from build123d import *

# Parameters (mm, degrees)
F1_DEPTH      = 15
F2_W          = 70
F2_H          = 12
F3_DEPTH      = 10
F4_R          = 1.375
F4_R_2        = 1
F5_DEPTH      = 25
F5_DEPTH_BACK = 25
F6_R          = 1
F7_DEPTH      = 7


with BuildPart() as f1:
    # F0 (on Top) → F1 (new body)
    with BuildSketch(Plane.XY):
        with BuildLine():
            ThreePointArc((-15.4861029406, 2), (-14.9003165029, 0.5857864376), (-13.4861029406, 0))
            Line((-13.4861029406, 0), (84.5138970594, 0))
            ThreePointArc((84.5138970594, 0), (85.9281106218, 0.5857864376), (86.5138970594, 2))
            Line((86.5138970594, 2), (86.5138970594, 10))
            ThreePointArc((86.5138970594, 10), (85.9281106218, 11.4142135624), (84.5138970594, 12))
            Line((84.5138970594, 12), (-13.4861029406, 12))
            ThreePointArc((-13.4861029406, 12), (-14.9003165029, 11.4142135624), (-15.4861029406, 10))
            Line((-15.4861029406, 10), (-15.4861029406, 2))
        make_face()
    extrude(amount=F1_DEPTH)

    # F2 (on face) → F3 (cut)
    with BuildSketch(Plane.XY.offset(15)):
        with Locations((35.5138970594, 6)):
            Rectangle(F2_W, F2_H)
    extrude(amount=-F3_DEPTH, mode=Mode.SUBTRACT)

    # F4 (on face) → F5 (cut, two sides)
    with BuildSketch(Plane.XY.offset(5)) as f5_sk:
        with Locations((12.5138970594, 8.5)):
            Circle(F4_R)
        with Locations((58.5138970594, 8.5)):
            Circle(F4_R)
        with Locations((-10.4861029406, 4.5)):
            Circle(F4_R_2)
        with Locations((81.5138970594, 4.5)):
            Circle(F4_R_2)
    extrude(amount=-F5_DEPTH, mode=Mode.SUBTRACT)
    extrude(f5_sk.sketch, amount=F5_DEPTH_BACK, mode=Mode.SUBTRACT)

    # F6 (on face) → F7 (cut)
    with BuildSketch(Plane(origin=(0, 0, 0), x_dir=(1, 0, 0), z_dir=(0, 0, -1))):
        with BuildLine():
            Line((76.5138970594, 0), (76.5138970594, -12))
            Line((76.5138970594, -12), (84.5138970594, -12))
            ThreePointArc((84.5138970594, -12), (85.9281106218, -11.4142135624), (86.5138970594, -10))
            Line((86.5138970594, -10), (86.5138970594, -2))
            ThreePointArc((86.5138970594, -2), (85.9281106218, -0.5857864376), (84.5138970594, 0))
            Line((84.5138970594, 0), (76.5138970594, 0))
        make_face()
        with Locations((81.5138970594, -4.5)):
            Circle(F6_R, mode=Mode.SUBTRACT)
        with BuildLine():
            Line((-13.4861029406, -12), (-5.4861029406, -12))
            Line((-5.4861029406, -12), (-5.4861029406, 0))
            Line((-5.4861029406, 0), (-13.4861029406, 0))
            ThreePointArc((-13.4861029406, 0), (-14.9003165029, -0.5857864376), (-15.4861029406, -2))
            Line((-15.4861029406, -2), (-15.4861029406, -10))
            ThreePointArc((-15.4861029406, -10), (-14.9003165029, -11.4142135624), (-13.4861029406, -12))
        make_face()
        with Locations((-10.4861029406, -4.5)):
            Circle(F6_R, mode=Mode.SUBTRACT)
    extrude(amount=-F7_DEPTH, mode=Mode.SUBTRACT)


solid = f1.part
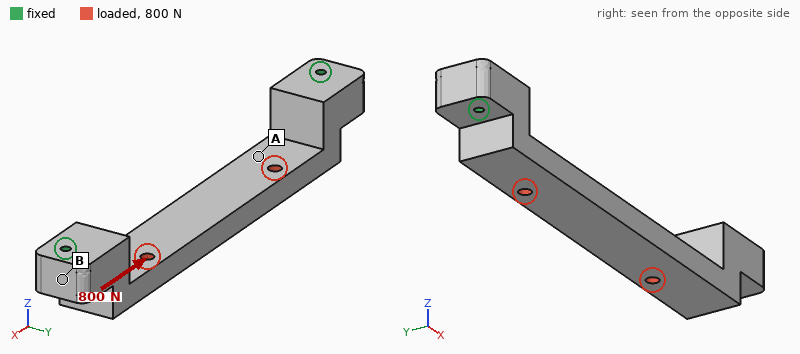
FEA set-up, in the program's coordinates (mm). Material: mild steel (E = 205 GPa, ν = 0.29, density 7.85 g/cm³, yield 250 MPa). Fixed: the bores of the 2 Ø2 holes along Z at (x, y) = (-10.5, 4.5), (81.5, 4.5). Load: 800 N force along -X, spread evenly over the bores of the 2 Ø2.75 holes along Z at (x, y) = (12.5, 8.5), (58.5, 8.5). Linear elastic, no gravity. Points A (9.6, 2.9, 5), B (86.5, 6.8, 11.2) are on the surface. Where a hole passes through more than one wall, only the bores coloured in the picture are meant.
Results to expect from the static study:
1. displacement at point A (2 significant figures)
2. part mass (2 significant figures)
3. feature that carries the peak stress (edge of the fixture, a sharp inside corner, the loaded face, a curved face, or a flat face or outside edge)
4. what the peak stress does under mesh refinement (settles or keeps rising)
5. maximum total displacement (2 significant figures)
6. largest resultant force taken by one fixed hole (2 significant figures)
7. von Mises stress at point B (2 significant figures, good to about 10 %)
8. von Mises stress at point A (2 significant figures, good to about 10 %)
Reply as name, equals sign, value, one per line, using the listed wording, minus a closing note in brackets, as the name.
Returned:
displacement at point A = 4.6 µm
part mass = 64 g
feature that carries the peak stress = edge of the fixture
what the peak stress does under mesh refinement = keeps rising
maximum total displacement = 5.2 µm
largest resultant force taken by one fixed hole = 400 N
von Mises stress at point B = 7.1 MPa
von Mises stress at point A = 17 MPa
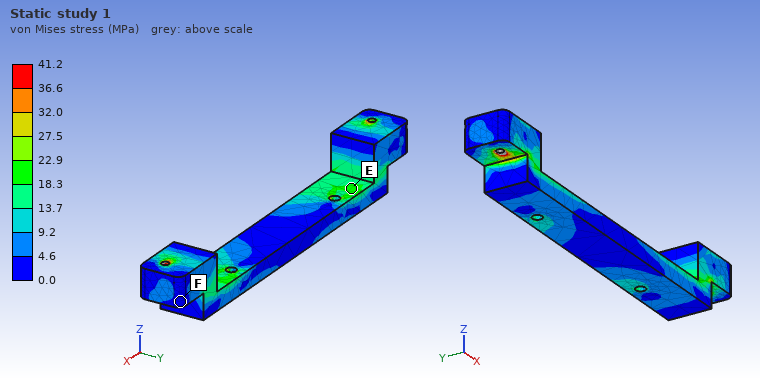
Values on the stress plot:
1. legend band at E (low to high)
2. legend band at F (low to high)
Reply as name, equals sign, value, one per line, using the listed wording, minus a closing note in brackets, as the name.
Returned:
legend band at E = 18.3 to 22.9 MPa
legend band at F = 0.0 to 4.6 MPa
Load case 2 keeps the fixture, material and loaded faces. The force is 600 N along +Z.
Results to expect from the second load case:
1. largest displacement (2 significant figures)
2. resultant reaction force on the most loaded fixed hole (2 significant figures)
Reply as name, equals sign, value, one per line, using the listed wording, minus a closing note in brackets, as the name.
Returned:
largest displacement = 27 µm
resultant reaction force on the most loaded fixed hole = 550 N
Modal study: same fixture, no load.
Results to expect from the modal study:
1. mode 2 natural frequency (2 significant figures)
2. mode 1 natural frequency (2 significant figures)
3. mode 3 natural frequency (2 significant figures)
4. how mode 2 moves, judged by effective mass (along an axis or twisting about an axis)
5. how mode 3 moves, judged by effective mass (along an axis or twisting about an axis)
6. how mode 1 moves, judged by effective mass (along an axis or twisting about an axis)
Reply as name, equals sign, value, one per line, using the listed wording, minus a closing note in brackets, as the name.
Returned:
mode 2 natural frequency = 4700 Hz
mode 1 natural frequency = 4100 Hz
mode 3 natural frequency = 8200 Hz
how mode 2 moves, judged by effective mass = along Y
how mode 3 moves, judged by effective mass = along X
how mode 1 moves, judged by effective mass = along Z
